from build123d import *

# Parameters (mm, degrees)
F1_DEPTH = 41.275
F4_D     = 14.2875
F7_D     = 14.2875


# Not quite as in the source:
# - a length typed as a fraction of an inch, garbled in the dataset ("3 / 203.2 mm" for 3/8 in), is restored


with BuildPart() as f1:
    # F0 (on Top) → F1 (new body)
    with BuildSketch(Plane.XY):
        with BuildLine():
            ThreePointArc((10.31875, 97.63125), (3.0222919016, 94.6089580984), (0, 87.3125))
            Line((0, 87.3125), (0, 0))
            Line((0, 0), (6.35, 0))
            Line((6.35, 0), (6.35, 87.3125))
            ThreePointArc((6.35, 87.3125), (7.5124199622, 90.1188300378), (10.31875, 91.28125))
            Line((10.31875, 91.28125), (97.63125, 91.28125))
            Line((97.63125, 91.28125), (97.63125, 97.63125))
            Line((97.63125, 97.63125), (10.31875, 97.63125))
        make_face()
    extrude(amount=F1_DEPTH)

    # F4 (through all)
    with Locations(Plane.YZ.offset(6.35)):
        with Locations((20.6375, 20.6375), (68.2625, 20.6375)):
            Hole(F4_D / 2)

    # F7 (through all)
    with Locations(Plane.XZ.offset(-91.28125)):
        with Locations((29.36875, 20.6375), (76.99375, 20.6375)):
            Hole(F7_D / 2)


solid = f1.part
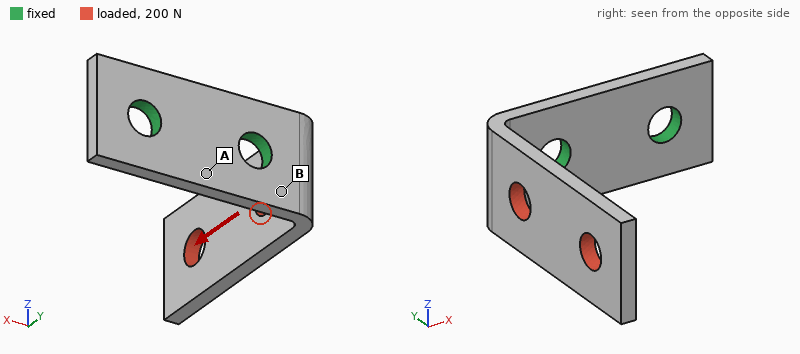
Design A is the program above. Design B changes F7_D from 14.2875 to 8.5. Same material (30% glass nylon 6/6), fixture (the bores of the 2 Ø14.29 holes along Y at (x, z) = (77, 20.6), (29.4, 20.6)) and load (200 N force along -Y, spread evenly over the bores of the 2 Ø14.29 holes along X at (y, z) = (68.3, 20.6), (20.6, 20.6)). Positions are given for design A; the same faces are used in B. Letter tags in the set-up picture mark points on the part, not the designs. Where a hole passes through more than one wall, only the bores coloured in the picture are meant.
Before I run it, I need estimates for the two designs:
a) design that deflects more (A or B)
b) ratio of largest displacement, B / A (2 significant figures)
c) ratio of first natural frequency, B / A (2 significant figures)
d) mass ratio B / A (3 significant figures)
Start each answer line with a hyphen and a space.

- B
- 1.4
- 0.96
- 1.03
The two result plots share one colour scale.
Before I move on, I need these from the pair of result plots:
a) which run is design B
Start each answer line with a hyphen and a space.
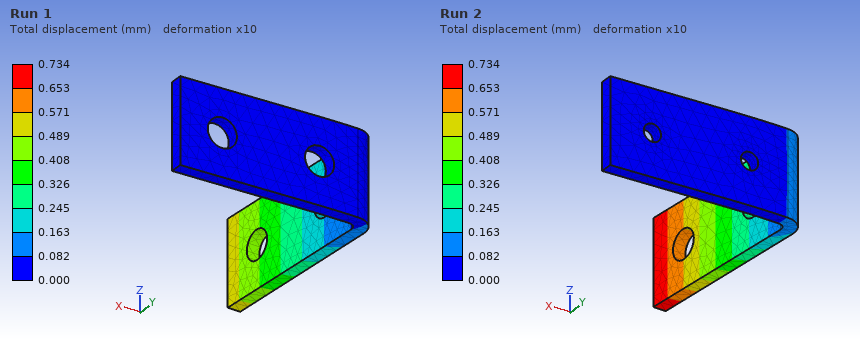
- Run 2
